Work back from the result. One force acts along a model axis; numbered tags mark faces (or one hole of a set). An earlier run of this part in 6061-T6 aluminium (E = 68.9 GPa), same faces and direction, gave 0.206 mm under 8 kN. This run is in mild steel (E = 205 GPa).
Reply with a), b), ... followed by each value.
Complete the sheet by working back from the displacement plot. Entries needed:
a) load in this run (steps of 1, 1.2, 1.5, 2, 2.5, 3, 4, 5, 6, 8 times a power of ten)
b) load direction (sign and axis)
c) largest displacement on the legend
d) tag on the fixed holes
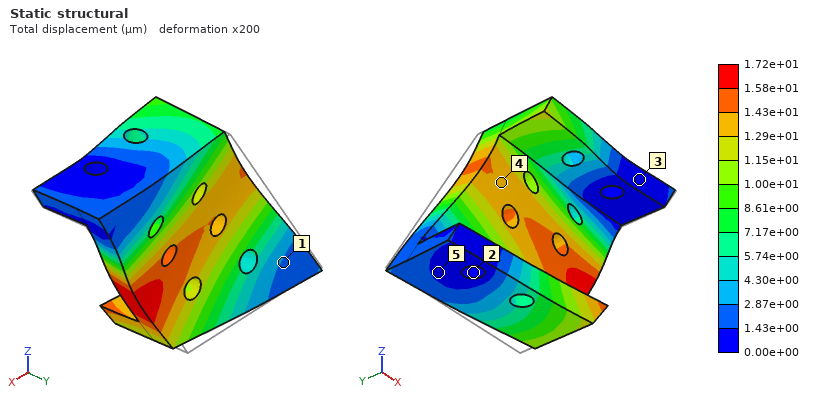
a) 2 kN
b) -Y
c) 1.72e+01 µm
d) 2
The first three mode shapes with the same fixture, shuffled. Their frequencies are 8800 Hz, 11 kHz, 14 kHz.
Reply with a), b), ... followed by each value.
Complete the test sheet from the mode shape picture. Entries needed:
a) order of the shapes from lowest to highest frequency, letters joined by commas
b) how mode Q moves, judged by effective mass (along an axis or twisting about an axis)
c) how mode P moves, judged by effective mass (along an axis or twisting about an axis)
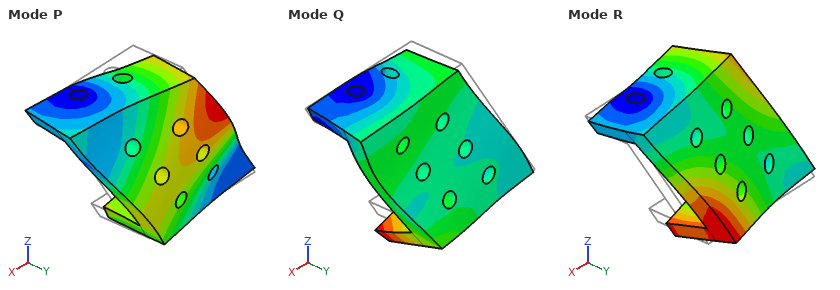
a) R, P, Q
b) along Z
c) along Y
